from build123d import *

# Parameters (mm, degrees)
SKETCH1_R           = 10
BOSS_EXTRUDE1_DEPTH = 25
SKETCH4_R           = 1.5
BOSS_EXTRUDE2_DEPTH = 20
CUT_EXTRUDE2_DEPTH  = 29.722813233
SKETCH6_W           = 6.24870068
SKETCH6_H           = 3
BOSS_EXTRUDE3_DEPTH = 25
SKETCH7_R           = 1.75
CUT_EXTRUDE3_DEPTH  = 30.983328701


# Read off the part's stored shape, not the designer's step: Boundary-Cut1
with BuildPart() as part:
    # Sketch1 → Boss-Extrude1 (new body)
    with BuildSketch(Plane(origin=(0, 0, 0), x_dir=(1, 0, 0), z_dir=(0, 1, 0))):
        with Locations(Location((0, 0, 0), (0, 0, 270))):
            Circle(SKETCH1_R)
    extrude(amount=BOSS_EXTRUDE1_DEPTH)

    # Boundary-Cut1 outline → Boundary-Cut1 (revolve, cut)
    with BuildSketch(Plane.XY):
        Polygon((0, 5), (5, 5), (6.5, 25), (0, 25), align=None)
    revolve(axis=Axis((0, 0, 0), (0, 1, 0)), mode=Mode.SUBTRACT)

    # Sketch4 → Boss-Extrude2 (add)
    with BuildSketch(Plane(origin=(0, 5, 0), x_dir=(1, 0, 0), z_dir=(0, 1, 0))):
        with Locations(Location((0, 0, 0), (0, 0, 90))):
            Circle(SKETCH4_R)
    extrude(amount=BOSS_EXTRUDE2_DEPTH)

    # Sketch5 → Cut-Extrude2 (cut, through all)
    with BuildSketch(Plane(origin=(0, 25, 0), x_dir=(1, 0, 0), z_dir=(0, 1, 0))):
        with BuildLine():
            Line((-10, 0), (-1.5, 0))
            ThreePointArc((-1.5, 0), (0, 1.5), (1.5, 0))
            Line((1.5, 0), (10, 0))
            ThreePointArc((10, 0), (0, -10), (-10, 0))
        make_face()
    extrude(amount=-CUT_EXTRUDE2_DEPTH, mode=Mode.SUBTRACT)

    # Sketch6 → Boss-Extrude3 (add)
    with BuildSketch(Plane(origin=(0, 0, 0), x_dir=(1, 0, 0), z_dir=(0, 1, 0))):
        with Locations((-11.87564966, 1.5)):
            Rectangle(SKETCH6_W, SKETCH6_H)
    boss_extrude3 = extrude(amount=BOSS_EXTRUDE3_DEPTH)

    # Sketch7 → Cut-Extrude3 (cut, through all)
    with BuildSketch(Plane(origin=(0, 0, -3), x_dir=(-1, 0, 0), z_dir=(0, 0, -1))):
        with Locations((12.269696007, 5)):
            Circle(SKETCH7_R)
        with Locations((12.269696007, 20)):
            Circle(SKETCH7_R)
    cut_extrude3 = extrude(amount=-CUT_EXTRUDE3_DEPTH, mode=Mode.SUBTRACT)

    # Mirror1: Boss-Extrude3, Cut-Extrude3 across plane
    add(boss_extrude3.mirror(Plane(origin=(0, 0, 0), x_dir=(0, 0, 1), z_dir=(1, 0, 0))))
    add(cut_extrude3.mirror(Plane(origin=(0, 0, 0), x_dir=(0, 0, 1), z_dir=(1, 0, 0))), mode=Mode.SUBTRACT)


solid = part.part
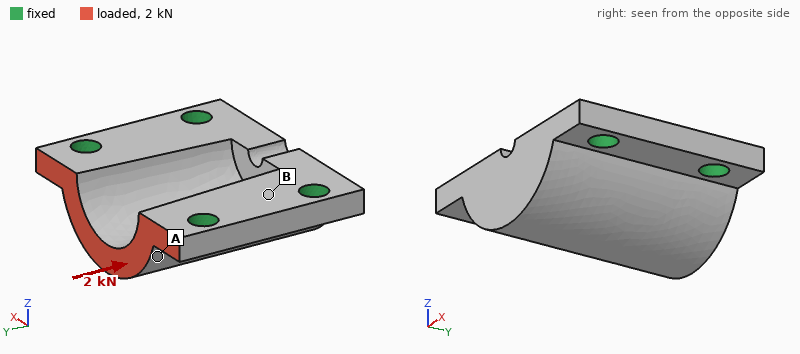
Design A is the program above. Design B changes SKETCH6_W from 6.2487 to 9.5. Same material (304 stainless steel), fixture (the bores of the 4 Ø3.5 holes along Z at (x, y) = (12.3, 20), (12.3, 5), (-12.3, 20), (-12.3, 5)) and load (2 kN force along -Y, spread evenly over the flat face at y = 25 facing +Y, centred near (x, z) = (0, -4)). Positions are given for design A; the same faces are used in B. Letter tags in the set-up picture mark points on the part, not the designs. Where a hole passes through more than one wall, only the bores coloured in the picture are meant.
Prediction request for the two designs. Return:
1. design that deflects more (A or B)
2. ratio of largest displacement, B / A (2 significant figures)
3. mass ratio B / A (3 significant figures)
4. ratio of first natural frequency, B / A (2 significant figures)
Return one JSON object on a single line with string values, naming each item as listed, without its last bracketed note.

{"design that deflects more": "A", "ratio of largest displacement, B / A": "0.91", "mass ratio B / A": "1.07", "ratio of first natural frequency, B / A": "1.0"}
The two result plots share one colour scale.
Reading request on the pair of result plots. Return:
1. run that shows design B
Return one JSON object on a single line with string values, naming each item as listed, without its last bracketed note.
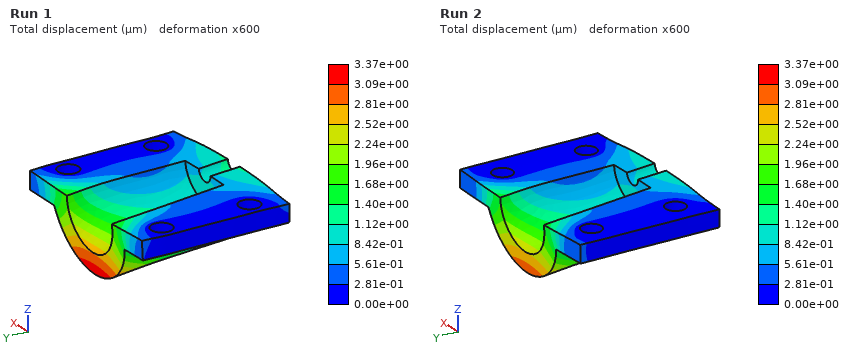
{"run that shows design B": "Run 2"}
